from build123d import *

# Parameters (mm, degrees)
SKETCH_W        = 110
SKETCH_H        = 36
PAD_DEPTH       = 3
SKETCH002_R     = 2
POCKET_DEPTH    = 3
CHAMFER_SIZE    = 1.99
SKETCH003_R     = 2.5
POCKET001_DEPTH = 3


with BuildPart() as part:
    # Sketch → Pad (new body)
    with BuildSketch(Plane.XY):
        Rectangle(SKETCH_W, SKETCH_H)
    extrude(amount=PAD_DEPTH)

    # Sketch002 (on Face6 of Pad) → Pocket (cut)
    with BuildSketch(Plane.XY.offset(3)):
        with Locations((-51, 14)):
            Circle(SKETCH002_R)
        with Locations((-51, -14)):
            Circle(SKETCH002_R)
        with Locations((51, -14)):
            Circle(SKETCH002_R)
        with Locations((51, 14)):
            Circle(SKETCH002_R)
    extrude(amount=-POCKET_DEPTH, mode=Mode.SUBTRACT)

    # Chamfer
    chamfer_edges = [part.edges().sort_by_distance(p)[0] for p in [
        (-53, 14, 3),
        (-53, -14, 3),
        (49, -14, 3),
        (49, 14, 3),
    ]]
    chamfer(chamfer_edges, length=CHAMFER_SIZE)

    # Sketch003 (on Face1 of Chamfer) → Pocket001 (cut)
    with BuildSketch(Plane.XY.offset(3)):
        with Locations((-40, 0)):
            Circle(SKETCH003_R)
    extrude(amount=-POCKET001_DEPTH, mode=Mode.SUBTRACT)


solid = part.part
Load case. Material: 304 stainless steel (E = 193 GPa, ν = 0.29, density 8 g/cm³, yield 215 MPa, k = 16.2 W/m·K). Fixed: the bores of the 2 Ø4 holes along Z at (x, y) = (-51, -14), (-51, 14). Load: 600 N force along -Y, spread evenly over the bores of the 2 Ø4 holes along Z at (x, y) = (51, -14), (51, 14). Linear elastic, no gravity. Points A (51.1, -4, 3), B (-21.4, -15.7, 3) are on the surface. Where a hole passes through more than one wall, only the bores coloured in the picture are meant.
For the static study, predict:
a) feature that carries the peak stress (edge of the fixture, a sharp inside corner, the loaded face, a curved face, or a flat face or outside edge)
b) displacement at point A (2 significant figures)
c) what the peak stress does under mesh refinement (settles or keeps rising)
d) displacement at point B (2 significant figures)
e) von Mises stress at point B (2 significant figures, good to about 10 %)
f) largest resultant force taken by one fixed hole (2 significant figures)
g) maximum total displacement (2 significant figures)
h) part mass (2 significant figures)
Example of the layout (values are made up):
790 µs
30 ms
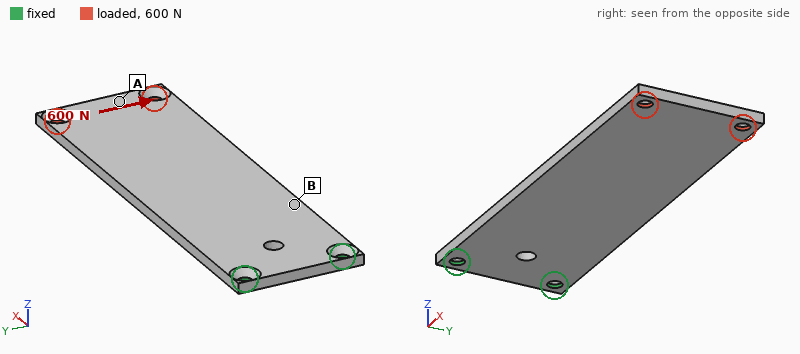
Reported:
edge of the fixture
0.12 mm
keeps rising
0.034 mm
56 MPa
2.1 kN
0.15 mm
92 g
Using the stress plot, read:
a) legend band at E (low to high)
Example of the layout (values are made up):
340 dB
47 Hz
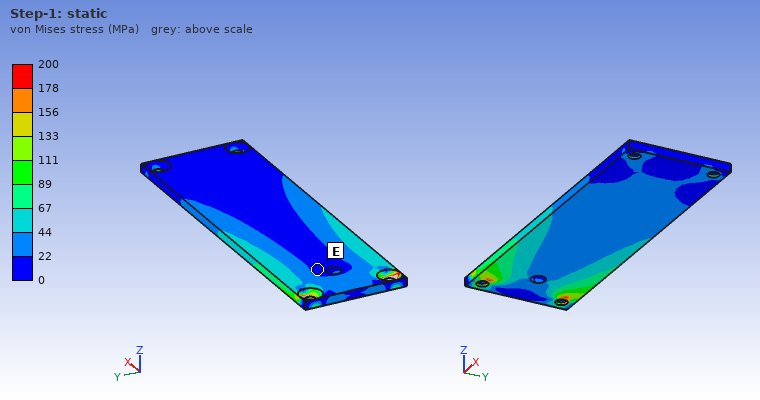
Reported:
0 to 22 MPa
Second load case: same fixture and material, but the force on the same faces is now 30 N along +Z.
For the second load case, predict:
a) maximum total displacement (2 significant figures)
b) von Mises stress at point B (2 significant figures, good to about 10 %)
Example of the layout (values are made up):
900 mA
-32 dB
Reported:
0.92 mm
41 MPa
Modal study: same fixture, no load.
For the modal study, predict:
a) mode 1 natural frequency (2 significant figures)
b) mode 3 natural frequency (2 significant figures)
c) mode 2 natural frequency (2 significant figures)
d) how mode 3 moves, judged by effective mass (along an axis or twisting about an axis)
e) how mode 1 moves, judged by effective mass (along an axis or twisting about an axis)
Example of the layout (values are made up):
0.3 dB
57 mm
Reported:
190 Hz
1300 Hz
1200 Hz
twisting about X
along Z
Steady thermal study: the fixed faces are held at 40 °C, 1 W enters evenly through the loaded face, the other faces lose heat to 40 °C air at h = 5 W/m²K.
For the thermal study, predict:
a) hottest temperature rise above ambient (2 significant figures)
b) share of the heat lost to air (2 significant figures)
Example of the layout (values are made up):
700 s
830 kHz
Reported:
40 K
64 %
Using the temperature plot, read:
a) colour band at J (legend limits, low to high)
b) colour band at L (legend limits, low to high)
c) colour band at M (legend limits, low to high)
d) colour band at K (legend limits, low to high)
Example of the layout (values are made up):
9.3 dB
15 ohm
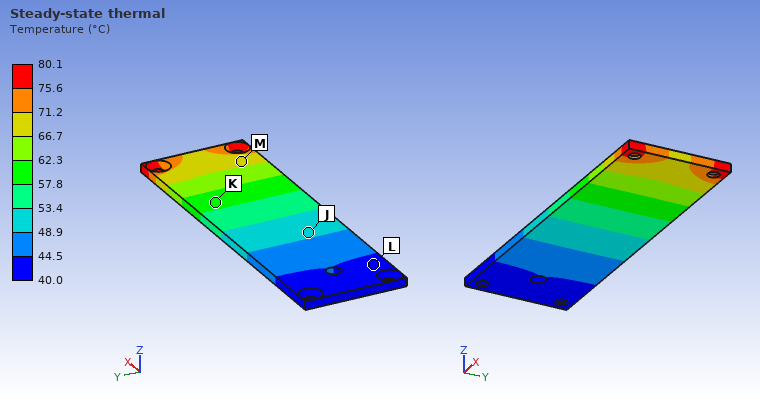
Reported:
48.9 to 53.4 °C
40.0 to 44.5 °C
66.7 to 71.2 °C
57.8 to 62.3 °C
